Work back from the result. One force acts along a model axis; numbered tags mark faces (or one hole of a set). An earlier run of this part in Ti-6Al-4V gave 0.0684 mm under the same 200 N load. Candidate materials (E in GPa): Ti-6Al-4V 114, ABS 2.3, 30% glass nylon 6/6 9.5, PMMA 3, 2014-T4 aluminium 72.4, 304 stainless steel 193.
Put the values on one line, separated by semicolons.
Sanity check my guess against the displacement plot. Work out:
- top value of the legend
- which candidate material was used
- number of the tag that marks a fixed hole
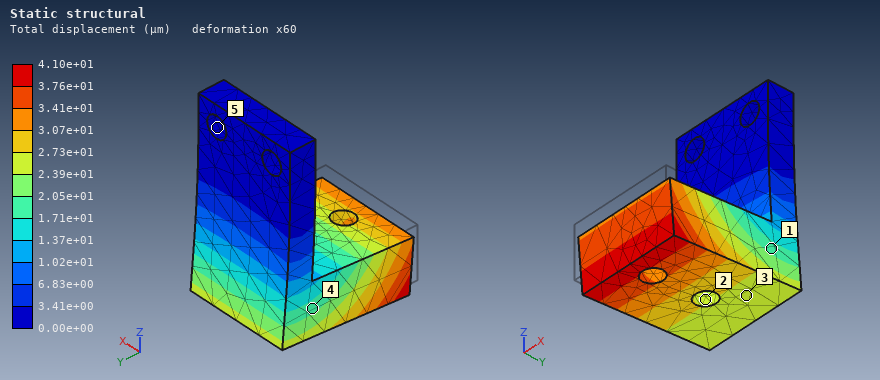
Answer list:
4.10e+01 µm; 304 stainless steel; 5
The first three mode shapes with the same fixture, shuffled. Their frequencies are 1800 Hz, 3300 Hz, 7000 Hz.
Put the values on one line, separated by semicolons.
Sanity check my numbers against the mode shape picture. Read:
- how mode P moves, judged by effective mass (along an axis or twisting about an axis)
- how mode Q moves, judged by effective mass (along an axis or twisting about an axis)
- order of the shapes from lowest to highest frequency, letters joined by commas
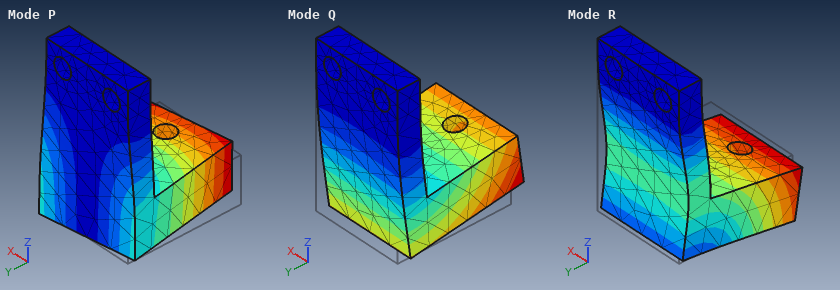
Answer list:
along X; along Y; Q, P, R
